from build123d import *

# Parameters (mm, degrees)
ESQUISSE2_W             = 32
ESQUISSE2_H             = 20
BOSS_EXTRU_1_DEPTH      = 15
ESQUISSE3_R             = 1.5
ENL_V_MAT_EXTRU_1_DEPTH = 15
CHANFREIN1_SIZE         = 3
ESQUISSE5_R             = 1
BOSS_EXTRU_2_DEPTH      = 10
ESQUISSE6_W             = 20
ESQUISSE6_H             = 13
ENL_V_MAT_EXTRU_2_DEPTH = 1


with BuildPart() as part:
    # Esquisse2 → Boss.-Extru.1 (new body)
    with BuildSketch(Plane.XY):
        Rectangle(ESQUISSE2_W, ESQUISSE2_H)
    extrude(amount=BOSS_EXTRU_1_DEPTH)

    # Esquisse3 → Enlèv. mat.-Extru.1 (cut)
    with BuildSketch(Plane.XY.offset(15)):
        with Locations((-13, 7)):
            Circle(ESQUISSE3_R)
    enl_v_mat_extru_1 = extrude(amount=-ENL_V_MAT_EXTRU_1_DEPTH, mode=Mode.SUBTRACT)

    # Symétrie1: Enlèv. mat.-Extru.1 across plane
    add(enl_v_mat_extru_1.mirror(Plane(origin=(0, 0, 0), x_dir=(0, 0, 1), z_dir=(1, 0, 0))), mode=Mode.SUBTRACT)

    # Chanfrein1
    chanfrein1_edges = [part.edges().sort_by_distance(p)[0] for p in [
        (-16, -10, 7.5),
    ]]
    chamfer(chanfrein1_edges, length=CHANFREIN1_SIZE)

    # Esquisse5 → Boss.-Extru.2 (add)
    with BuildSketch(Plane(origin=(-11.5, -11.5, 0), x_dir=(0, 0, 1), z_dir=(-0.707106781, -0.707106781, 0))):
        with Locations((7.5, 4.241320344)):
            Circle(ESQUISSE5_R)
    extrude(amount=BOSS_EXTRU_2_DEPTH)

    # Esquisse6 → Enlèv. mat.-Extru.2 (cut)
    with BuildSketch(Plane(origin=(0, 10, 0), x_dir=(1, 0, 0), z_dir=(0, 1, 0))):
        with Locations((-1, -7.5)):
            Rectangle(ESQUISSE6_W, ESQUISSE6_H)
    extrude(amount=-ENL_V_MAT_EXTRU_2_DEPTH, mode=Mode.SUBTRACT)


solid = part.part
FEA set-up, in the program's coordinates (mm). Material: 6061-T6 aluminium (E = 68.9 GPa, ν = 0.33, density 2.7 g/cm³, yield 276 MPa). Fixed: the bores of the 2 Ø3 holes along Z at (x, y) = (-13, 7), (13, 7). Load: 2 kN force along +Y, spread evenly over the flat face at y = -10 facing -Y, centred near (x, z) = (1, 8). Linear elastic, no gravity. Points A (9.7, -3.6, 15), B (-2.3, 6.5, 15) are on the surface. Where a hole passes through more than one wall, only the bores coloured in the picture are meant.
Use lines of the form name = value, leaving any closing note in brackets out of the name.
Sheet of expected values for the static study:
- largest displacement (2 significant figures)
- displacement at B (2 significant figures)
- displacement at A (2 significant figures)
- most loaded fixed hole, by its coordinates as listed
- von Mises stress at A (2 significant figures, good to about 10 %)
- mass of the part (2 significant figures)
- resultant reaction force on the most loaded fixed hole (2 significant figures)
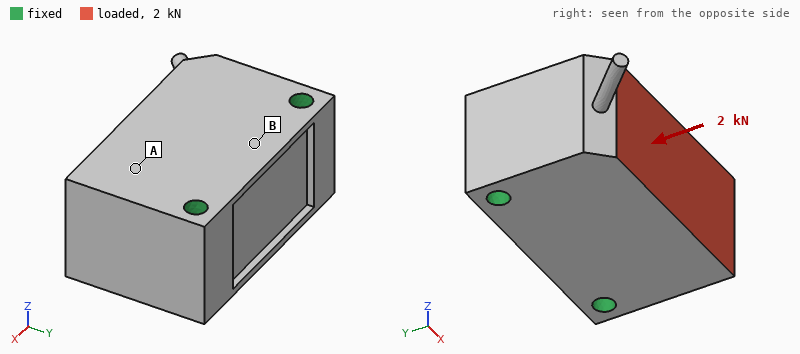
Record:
largest displacement = 2.0 µm
displacement at B = 1.4 µm
displacement at A = 1.3 µm
most loaded fixed hole, by its coordinates as listed = (13, 7)
von Mises stress at A = 5.6 MPa
mass of the part = 25 g
resultant reaction force on the most loaded fixed hole = 1.2 kN
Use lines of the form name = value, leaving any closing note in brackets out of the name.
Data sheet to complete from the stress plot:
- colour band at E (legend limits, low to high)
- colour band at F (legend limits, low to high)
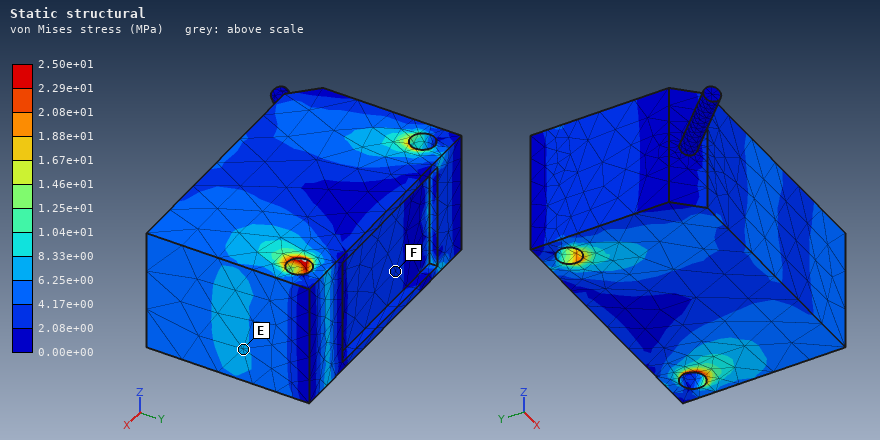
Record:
colour band at E = 6.25e+00 to 8.33e+00 MPa
colour band at F = 2.08e+00 to 4.17e+00 MPa
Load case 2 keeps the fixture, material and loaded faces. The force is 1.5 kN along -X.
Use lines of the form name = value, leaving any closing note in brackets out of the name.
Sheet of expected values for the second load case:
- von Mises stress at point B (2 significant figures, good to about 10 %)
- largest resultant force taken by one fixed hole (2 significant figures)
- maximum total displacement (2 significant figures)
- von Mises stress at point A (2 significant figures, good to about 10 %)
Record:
von Mises stress at point B = 2.3 MPa
largest resultant force taken by one fixed hole = 1.2 kN
maximum total displacement = 4.8 µm
von Mises stress at point A = 5.8 MPa
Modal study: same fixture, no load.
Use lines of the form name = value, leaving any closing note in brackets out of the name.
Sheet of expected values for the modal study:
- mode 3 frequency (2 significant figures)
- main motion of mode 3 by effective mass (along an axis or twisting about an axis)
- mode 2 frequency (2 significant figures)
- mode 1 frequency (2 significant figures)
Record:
mode 3 frequency = 21 kHz
main motion of mode 3 by effective mass = along Z
mode 2 frequency = 13 kHz
mode 1 frequency = 13 kHz
